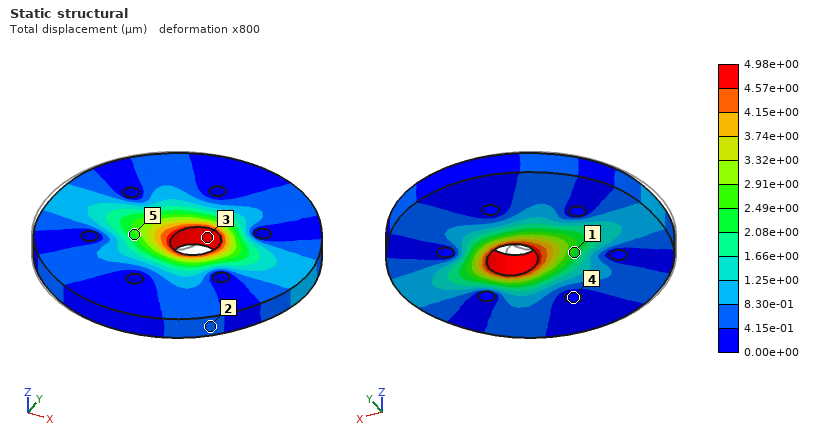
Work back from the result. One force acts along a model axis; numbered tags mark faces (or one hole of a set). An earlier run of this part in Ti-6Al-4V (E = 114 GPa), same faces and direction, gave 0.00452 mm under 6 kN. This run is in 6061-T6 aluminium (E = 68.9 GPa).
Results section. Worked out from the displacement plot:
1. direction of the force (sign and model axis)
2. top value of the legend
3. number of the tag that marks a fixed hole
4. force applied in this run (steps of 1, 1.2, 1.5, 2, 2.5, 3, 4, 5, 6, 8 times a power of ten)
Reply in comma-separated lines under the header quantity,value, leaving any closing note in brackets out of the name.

quantity,value
direction of the force,+X
top value of the legend,4.98e+00 µm
number of the tag that marks a fixed hole,4
force applied in this run,4 kN
